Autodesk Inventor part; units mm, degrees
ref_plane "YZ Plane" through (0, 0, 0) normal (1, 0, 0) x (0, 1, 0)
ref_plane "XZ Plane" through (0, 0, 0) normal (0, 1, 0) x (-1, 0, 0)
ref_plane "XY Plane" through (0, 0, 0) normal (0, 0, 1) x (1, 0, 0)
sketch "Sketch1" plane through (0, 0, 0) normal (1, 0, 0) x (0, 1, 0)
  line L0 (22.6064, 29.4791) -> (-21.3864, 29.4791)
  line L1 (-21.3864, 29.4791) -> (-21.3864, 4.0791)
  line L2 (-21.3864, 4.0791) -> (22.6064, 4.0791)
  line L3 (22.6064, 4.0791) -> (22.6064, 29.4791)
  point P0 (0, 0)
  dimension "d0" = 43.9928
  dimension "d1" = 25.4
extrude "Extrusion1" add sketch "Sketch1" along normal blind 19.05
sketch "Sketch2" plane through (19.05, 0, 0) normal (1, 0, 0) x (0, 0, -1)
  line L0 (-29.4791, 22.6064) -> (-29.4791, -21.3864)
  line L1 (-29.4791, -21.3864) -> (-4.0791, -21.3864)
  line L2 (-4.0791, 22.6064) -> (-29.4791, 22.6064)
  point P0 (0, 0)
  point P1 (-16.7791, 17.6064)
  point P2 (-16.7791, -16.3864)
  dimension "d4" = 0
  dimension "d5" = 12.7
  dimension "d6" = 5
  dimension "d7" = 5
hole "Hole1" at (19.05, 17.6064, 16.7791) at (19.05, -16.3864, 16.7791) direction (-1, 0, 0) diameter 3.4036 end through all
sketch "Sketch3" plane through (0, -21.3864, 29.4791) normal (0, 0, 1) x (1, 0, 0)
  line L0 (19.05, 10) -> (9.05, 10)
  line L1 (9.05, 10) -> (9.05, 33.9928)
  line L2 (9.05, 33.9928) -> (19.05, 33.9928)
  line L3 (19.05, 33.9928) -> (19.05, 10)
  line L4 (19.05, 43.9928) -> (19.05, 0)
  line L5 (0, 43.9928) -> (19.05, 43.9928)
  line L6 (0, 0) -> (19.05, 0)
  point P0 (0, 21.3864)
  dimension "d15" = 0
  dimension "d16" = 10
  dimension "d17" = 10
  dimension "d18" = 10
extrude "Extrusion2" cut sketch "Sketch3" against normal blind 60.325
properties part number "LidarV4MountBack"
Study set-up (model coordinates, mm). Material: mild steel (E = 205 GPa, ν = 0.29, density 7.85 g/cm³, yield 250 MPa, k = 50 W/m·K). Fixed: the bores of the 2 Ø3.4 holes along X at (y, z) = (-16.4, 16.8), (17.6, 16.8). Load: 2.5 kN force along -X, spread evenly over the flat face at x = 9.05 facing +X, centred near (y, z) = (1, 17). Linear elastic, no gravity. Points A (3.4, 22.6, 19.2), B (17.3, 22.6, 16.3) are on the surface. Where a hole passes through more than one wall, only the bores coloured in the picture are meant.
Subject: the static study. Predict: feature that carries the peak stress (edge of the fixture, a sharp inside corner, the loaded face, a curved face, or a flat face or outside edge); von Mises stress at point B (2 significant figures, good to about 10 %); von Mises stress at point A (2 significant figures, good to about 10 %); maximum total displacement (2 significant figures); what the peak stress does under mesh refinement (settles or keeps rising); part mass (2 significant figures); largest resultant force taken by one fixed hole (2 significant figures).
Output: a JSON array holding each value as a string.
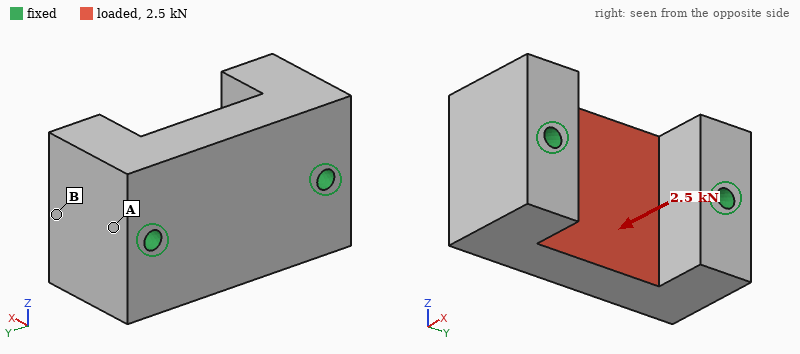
["edge of the fixture", "10 MPa", "3.8 MPa", "2.1 µm", "keeps rising", "120 g", "1.3 kN"]
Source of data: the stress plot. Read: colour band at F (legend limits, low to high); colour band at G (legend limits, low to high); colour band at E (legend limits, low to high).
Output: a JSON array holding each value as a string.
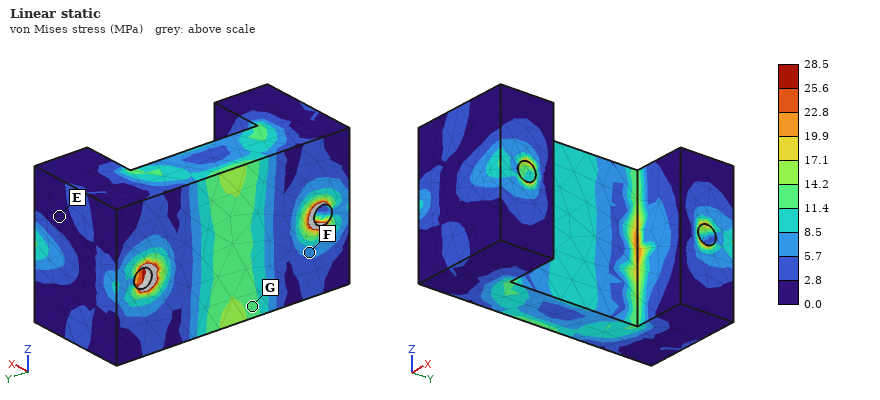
["5.7 to 8.5 MPa", "11.4 to 14.2 MPa", "0.0 to 2.8 MPa"]
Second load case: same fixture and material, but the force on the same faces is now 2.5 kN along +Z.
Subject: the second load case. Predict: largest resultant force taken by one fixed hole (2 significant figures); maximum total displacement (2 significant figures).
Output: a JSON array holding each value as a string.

["1.3 kN", "2.3 µm"]
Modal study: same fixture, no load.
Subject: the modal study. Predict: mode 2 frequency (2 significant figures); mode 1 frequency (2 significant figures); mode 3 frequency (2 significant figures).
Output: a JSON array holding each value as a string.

["29 kHz", "29 kHz", "34 kHz"]
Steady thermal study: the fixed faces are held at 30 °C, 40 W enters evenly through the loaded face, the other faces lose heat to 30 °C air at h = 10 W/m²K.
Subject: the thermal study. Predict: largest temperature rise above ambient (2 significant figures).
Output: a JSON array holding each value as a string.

["25 K"]
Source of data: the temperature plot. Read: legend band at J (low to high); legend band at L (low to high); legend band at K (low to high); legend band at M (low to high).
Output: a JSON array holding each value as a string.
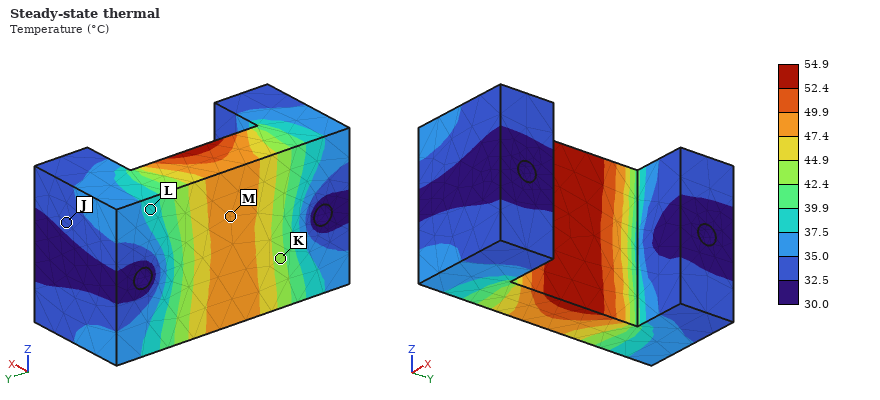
["32.5 to 35.0 °C", "37.5 to 39.9 °C", "42.4 to 44.9 °C", "47.4 to 49.9 °C"]
